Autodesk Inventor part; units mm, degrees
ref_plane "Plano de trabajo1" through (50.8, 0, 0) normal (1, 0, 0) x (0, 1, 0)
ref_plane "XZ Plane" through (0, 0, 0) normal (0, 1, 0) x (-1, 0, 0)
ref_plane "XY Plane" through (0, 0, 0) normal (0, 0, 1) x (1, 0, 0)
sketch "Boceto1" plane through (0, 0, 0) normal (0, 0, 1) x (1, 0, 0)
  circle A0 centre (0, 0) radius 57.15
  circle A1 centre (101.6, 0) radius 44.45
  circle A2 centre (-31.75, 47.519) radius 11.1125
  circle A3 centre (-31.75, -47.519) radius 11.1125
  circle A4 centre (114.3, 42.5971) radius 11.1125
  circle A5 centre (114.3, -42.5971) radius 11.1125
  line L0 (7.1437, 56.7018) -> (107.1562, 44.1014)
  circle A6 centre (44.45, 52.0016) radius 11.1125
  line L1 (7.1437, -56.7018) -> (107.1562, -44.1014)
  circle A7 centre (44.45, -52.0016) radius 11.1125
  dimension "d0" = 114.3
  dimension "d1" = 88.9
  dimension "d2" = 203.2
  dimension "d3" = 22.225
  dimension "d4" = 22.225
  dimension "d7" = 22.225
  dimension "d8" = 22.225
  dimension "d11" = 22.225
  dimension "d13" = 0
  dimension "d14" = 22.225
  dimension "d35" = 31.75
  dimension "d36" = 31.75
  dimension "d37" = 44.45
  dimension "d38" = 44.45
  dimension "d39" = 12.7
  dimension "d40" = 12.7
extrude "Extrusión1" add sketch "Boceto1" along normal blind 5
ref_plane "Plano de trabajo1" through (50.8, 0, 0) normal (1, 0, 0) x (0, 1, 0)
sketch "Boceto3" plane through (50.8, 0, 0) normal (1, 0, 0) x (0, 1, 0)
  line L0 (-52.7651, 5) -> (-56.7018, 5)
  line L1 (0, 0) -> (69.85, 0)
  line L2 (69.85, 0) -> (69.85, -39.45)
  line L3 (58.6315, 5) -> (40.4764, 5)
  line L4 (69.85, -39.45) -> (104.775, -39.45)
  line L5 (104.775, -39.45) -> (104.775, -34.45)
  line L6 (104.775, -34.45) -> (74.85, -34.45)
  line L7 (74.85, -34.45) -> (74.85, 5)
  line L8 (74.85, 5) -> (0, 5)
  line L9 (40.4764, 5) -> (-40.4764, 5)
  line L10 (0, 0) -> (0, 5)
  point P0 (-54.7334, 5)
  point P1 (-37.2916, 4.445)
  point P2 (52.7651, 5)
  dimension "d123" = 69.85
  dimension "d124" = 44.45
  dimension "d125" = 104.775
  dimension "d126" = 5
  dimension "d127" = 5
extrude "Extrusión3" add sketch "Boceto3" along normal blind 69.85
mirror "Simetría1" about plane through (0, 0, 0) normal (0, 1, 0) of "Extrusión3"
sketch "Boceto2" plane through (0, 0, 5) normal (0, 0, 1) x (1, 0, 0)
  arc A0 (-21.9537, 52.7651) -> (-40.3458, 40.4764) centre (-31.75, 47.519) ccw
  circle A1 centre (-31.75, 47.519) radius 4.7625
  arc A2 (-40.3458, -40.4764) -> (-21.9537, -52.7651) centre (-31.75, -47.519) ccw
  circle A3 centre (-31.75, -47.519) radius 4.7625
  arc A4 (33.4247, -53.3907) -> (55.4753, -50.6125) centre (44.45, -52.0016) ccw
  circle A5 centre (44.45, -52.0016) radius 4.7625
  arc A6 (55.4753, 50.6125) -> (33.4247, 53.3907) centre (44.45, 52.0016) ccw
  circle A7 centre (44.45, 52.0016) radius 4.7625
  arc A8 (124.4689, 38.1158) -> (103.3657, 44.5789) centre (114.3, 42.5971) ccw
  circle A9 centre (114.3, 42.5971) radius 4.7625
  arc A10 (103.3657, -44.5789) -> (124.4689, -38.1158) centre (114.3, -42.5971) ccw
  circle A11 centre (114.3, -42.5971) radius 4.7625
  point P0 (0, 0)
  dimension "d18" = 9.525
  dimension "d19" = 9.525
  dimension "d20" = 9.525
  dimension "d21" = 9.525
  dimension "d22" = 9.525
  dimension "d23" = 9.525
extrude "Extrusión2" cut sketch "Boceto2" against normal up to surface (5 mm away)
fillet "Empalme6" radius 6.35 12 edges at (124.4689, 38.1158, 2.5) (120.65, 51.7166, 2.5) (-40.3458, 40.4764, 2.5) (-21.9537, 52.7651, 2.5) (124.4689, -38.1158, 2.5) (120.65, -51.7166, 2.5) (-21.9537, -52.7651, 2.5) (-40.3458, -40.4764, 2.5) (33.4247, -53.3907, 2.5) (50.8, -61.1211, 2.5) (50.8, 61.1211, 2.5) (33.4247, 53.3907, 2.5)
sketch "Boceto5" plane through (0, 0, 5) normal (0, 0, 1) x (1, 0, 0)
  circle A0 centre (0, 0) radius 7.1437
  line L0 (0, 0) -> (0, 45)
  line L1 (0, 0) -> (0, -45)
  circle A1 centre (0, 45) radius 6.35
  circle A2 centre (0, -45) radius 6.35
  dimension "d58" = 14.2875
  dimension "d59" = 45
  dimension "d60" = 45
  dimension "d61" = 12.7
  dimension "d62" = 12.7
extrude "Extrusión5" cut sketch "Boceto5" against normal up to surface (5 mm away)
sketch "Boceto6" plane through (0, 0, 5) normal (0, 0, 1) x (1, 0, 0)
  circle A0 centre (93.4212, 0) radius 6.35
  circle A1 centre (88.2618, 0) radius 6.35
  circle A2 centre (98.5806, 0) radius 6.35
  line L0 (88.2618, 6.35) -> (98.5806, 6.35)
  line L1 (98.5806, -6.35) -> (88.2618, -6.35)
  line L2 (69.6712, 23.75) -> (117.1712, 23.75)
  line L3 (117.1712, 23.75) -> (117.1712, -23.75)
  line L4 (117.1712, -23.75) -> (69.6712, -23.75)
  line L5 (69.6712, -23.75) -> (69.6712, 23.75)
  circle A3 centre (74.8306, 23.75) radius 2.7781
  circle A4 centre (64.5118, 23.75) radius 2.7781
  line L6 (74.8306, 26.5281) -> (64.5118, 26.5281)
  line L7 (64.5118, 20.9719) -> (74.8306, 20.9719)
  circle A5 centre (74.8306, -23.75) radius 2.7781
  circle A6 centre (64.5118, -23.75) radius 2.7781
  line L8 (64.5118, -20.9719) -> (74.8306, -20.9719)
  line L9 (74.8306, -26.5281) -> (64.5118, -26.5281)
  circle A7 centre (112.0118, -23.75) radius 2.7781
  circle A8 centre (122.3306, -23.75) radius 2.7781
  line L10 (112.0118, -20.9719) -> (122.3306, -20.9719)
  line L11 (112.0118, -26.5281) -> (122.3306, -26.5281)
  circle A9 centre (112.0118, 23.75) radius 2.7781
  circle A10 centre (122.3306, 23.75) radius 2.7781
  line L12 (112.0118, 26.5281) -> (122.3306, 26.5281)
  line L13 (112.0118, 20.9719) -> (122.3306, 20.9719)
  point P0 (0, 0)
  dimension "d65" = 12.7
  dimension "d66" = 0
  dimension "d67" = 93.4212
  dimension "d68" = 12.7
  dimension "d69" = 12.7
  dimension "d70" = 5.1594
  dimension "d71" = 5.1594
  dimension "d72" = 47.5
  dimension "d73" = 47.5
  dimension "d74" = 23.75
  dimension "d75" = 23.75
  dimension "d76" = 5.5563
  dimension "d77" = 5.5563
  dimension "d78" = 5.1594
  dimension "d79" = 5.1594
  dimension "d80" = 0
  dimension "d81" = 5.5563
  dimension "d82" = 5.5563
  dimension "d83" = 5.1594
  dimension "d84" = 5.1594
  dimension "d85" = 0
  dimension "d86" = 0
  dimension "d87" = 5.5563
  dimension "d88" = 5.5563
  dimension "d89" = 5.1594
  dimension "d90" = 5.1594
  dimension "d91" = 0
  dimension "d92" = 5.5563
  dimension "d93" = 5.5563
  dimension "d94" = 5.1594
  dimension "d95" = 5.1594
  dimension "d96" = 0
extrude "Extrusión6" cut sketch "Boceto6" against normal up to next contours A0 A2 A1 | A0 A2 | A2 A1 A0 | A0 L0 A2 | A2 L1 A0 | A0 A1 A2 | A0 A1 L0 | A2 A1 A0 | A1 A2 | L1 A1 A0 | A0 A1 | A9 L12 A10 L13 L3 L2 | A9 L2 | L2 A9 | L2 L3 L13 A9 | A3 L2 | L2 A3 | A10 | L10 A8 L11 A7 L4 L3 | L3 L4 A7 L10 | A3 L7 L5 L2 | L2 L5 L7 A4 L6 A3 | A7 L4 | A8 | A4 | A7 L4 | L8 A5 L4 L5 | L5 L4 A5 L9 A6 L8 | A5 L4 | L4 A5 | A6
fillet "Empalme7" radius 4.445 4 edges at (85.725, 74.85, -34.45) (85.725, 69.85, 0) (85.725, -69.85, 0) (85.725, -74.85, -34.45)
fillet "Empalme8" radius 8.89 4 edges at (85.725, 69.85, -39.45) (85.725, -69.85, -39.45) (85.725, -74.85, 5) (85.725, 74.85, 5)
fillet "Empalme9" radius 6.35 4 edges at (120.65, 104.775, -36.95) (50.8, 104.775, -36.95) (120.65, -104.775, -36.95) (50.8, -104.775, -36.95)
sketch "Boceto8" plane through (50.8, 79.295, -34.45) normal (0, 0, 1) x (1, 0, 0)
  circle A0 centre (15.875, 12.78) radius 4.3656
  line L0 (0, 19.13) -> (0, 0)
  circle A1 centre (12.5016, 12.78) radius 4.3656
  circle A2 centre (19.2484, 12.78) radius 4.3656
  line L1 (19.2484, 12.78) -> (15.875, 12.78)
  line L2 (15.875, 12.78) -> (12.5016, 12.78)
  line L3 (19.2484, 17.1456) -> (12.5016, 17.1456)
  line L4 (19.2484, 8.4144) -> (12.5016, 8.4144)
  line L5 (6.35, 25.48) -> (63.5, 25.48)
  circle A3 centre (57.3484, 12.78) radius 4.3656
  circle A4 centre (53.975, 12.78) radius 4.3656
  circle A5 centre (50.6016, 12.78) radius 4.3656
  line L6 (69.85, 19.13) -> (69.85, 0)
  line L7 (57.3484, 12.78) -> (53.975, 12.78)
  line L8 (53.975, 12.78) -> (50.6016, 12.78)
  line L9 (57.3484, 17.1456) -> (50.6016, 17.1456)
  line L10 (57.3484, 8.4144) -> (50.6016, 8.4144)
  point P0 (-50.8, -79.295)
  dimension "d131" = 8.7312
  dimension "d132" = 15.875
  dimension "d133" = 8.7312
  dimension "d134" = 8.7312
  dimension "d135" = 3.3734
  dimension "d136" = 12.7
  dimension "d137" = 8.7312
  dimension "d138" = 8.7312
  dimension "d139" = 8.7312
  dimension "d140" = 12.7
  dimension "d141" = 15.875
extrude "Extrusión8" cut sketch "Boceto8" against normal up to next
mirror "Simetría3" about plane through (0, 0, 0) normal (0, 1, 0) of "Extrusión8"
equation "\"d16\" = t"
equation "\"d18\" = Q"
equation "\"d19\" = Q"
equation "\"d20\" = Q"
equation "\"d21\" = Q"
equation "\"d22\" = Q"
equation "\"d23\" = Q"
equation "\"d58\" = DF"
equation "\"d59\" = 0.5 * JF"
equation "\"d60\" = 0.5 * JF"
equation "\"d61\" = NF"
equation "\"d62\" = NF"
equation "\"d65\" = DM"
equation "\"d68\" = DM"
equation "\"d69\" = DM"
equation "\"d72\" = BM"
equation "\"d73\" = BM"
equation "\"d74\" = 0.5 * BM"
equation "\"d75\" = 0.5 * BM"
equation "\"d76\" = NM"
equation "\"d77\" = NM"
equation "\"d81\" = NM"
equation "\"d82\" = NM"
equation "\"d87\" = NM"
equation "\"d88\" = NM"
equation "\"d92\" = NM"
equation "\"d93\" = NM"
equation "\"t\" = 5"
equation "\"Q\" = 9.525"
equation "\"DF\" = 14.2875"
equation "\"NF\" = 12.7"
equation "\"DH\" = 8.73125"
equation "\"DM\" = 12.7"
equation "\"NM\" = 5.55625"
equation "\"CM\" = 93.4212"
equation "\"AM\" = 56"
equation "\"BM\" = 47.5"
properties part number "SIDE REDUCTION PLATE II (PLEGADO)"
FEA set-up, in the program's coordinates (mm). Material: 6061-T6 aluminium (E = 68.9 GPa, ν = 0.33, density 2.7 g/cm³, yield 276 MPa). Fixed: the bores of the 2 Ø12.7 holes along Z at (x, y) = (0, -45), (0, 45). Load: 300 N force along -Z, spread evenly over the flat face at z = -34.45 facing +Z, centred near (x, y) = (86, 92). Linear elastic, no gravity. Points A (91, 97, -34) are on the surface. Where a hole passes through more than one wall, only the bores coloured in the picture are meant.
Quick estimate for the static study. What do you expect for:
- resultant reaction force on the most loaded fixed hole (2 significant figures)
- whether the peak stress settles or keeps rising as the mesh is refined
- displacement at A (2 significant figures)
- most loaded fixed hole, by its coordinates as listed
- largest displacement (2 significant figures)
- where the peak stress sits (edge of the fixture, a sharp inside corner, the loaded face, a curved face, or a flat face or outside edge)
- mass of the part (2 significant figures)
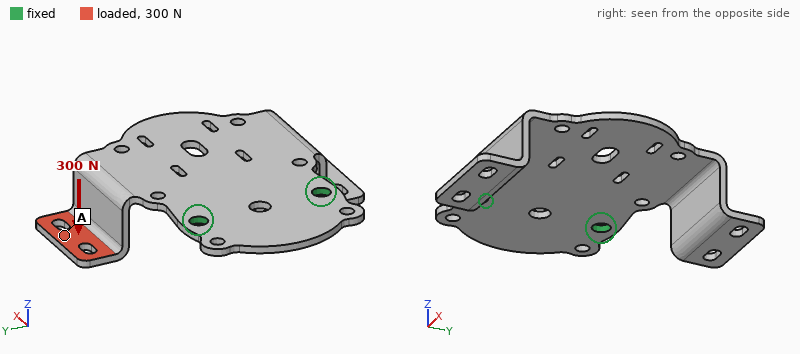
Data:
450 N
keeps rising
2.4 mm
(0, 45)
3.1 mm
edge of the fixture
410 g
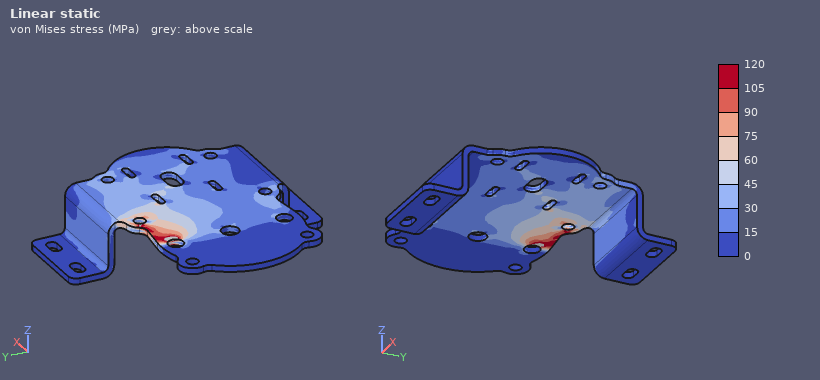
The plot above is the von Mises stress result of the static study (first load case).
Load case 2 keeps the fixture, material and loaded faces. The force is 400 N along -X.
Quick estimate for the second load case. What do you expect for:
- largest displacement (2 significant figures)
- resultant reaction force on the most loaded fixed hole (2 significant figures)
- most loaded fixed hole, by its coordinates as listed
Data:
1.8 mm
610 N
(0, 45)
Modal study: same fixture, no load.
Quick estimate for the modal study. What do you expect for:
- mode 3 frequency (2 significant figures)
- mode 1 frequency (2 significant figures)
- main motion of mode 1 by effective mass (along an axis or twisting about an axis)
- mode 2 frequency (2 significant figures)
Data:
450 Hz
160 Hz
along Z
250 Hz
